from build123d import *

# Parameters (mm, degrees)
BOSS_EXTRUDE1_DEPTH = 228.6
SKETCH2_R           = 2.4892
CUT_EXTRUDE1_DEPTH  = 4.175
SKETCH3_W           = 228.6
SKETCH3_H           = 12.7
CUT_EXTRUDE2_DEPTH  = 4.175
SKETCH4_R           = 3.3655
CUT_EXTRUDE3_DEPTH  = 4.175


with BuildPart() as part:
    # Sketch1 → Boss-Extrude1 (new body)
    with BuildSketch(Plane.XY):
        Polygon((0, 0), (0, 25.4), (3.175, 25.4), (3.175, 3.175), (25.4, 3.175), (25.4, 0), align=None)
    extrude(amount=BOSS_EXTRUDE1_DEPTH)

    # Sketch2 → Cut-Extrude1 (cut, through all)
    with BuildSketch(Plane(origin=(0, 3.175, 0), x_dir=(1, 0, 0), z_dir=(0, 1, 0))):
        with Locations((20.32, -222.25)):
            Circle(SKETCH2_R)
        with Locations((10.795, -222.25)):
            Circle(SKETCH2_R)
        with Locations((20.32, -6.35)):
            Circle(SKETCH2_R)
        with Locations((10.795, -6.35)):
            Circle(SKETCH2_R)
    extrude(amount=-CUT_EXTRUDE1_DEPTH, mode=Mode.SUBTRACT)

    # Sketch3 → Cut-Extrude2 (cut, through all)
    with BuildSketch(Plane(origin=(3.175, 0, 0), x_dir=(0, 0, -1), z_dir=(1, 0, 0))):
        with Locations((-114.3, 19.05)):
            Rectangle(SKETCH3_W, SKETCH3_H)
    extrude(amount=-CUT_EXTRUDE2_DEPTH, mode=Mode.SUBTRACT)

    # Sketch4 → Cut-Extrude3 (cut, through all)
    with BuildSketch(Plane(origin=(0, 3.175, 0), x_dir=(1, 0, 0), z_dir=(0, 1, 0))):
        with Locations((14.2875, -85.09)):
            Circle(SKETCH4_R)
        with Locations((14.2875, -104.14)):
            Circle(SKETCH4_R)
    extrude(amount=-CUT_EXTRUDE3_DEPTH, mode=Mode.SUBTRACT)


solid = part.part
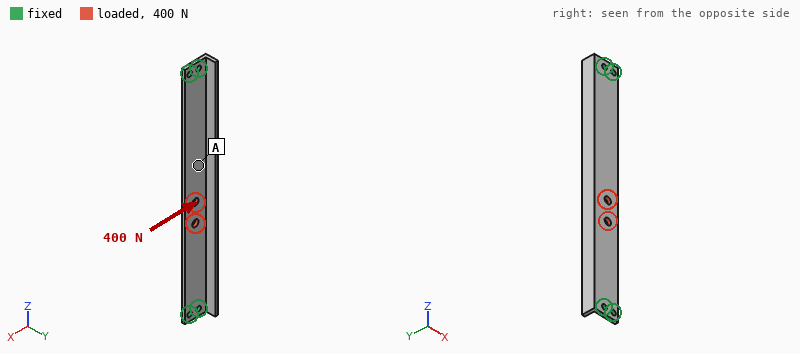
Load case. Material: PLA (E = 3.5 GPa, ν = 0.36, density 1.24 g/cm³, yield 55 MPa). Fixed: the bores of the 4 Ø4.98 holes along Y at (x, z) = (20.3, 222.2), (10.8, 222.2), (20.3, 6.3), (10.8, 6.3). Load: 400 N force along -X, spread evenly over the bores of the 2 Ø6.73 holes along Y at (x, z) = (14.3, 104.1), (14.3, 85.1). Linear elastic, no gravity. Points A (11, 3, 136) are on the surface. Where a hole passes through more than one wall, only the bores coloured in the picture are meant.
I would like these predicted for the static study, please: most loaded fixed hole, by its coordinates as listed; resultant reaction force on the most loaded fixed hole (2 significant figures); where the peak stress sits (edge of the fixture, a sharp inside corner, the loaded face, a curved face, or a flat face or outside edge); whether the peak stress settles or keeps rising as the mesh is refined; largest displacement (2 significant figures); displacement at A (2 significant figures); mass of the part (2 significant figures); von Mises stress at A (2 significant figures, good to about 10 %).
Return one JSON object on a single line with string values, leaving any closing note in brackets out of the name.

{"most loaded fixed hole, by its coordinates as listed": "(20.3, 6.3)", "resultant reaction force on the most loaded fixed hole": "810 N", "where the peak stress sits": "edge of the fixture", "whether the peak stress settles or keeps rising as the mesh is refined": "keeps rising", "largest displacement": "2.2 mm", "displacement at A": "1.7 mm", "mass of the part": "31 g", "von Mises stress at A": "4.9 MPa"}
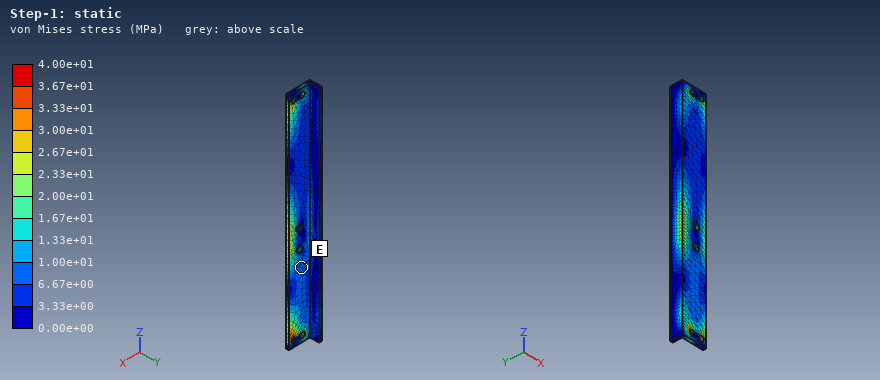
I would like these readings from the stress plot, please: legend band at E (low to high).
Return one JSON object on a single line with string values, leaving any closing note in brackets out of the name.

{"legend band at E": "6.67e+00 to 1.00e+01 MPa"}
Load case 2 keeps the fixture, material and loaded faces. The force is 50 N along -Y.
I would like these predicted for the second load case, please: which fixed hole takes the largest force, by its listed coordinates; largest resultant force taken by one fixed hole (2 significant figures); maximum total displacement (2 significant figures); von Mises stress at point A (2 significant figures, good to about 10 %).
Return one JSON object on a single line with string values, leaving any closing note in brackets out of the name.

{"which fixed hole takes the largest force, by its listed coordinates": "(10.8, 6.3)", "largest resultant force taken by one fixed hole": "110 N", "maximum total displacement": "2.4 mm", "von Mises stress at point A": "3.5 MPa"}
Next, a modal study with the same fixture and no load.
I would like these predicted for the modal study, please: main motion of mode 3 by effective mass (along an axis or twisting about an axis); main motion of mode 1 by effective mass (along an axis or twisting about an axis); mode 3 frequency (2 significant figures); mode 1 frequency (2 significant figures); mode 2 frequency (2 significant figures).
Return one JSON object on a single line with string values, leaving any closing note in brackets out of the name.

{"main motion of mode 3 by effective mass": "twisting about X", "main motion of mode 1 by effective mass": "along Y", "mode 3 frequency": "650 Hz", "mode 1 frequency": "240 Hz", "mode 2 frequency": "500 Hz"}
